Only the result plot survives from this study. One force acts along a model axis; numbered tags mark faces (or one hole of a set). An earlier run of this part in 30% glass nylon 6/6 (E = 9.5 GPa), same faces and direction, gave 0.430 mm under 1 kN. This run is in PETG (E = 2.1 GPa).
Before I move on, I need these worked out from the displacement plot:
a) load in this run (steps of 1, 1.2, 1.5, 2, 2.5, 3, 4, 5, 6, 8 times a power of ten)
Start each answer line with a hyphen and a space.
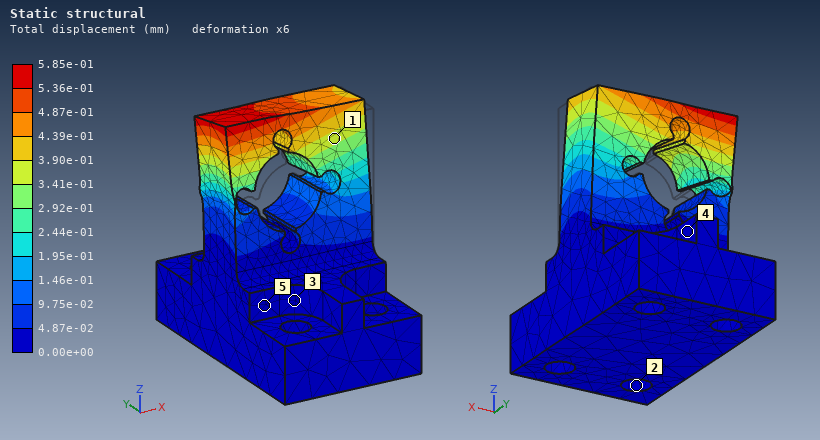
- 300 N
